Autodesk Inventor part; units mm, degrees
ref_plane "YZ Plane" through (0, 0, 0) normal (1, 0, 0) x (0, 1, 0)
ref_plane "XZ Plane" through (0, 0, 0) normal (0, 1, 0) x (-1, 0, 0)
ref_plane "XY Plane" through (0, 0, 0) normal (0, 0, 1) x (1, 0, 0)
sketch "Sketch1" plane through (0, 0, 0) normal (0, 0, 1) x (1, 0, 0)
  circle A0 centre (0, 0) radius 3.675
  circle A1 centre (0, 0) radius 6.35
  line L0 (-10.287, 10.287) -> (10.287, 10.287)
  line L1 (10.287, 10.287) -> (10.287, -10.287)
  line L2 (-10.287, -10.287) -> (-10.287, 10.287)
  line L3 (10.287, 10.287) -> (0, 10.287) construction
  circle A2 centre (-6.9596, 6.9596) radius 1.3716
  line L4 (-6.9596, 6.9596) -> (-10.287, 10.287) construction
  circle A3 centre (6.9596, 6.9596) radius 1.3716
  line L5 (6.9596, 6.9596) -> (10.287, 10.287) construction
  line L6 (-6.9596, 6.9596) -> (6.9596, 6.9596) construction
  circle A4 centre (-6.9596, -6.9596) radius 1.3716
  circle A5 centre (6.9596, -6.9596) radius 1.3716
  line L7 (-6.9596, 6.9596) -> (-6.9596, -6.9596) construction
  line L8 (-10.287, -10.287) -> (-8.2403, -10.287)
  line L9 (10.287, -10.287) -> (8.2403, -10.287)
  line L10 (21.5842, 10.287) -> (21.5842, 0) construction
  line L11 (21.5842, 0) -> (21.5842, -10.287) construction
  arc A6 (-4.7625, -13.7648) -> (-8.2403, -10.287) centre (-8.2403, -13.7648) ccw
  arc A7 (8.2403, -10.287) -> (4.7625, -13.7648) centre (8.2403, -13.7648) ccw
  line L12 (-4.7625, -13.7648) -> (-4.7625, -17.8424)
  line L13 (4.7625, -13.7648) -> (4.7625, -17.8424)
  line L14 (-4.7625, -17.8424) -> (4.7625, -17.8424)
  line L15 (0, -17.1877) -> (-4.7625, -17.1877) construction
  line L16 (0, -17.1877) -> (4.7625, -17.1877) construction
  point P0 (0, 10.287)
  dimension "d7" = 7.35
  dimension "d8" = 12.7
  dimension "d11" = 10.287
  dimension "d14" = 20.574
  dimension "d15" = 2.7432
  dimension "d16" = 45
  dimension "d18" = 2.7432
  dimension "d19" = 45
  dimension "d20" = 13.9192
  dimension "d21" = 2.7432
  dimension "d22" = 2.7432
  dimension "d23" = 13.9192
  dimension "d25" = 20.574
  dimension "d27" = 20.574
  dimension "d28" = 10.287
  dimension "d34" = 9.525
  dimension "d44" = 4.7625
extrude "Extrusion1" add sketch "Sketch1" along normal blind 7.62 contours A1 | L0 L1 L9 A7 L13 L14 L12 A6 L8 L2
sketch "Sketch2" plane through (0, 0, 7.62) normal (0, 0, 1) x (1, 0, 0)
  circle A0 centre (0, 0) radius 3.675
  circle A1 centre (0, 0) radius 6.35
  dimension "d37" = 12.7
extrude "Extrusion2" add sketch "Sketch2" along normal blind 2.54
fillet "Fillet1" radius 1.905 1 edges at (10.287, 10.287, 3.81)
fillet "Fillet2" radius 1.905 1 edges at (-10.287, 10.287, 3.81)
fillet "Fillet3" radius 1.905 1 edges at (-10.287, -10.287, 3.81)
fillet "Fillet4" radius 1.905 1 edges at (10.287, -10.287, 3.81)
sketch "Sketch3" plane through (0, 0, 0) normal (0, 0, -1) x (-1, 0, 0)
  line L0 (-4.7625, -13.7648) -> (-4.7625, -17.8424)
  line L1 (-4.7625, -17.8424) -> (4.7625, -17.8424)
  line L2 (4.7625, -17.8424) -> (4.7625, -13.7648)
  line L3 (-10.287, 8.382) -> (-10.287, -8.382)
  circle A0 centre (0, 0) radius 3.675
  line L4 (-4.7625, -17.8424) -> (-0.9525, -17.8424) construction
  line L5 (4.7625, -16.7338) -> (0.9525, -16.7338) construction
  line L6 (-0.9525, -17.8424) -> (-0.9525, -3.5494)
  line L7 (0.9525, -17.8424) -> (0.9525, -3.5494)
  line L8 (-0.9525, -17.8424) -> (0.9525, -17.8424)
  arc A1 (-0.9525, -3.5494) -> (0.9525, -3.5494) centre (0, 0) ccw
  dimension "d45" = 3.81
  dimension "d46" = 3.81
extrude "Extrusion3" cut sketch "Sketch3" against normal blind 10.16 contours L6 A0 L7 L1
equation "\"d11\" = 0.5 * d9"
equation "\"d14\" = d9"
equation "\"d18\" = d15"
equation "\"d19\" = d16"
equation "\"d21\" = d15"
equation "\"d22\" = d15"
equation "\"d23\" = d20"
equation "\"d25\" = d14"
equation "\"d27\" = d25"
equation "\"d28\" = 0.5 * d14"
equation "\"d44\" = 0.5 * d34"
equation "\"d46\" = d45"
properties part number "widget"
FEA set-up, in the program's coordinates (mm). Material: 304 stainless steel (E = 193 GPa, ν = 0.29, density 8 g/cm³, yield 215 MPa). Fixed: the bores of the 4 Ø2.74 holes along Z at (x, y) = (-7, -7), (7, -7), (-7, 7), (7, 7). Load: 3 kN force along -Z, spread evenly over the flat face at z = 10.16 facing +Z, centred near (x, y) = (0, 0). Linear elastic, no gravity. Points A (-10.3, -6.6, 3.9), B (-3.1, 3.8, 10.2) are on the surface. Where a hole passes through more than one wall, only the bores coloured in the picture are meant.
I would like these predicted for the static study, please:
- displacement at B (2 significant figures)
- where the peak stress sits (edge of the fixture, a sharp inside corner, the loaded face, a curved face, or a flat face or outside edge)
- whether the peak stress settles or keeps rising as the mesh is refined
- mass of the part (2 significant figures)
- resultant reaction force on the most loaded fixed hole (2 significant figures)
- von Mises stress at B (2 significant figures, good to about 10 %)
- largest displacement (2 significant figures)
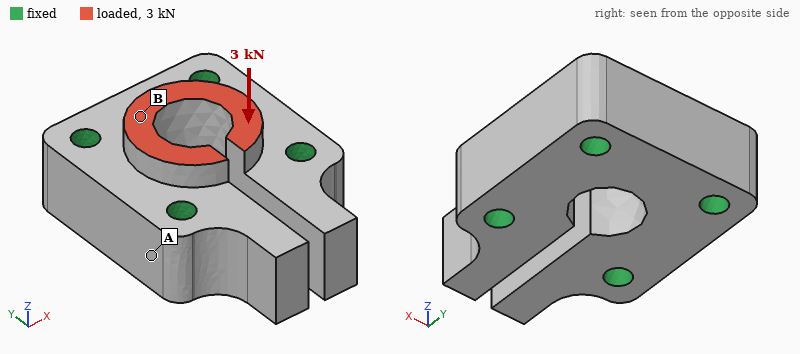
1.7 µm
edge of the fixture
keeps rising
26 g
800 N
32 MPa
2.7 µm
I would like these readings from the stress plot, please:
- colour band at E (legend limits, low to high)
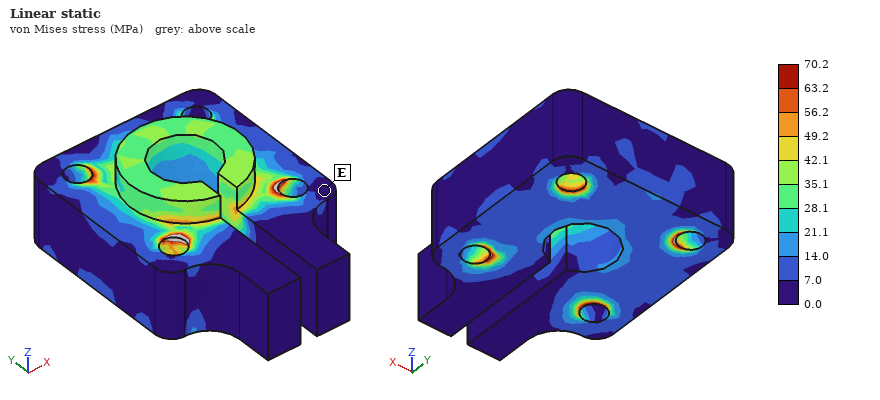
0.0 to 7.0 MPa
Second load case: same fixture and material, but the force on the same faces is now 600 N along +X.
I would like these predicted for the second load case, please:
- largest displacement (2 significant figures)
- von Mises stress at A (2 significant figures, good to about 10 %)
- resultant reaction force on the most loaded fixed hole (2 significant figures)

1.9 µm
3.1 MPa
230 N
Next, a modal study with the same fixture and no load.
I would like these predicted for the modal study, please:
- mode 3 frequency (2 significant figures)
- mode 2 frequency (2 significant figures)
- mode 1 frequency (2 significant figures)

41 kHz
35 kHz
35 kHz
